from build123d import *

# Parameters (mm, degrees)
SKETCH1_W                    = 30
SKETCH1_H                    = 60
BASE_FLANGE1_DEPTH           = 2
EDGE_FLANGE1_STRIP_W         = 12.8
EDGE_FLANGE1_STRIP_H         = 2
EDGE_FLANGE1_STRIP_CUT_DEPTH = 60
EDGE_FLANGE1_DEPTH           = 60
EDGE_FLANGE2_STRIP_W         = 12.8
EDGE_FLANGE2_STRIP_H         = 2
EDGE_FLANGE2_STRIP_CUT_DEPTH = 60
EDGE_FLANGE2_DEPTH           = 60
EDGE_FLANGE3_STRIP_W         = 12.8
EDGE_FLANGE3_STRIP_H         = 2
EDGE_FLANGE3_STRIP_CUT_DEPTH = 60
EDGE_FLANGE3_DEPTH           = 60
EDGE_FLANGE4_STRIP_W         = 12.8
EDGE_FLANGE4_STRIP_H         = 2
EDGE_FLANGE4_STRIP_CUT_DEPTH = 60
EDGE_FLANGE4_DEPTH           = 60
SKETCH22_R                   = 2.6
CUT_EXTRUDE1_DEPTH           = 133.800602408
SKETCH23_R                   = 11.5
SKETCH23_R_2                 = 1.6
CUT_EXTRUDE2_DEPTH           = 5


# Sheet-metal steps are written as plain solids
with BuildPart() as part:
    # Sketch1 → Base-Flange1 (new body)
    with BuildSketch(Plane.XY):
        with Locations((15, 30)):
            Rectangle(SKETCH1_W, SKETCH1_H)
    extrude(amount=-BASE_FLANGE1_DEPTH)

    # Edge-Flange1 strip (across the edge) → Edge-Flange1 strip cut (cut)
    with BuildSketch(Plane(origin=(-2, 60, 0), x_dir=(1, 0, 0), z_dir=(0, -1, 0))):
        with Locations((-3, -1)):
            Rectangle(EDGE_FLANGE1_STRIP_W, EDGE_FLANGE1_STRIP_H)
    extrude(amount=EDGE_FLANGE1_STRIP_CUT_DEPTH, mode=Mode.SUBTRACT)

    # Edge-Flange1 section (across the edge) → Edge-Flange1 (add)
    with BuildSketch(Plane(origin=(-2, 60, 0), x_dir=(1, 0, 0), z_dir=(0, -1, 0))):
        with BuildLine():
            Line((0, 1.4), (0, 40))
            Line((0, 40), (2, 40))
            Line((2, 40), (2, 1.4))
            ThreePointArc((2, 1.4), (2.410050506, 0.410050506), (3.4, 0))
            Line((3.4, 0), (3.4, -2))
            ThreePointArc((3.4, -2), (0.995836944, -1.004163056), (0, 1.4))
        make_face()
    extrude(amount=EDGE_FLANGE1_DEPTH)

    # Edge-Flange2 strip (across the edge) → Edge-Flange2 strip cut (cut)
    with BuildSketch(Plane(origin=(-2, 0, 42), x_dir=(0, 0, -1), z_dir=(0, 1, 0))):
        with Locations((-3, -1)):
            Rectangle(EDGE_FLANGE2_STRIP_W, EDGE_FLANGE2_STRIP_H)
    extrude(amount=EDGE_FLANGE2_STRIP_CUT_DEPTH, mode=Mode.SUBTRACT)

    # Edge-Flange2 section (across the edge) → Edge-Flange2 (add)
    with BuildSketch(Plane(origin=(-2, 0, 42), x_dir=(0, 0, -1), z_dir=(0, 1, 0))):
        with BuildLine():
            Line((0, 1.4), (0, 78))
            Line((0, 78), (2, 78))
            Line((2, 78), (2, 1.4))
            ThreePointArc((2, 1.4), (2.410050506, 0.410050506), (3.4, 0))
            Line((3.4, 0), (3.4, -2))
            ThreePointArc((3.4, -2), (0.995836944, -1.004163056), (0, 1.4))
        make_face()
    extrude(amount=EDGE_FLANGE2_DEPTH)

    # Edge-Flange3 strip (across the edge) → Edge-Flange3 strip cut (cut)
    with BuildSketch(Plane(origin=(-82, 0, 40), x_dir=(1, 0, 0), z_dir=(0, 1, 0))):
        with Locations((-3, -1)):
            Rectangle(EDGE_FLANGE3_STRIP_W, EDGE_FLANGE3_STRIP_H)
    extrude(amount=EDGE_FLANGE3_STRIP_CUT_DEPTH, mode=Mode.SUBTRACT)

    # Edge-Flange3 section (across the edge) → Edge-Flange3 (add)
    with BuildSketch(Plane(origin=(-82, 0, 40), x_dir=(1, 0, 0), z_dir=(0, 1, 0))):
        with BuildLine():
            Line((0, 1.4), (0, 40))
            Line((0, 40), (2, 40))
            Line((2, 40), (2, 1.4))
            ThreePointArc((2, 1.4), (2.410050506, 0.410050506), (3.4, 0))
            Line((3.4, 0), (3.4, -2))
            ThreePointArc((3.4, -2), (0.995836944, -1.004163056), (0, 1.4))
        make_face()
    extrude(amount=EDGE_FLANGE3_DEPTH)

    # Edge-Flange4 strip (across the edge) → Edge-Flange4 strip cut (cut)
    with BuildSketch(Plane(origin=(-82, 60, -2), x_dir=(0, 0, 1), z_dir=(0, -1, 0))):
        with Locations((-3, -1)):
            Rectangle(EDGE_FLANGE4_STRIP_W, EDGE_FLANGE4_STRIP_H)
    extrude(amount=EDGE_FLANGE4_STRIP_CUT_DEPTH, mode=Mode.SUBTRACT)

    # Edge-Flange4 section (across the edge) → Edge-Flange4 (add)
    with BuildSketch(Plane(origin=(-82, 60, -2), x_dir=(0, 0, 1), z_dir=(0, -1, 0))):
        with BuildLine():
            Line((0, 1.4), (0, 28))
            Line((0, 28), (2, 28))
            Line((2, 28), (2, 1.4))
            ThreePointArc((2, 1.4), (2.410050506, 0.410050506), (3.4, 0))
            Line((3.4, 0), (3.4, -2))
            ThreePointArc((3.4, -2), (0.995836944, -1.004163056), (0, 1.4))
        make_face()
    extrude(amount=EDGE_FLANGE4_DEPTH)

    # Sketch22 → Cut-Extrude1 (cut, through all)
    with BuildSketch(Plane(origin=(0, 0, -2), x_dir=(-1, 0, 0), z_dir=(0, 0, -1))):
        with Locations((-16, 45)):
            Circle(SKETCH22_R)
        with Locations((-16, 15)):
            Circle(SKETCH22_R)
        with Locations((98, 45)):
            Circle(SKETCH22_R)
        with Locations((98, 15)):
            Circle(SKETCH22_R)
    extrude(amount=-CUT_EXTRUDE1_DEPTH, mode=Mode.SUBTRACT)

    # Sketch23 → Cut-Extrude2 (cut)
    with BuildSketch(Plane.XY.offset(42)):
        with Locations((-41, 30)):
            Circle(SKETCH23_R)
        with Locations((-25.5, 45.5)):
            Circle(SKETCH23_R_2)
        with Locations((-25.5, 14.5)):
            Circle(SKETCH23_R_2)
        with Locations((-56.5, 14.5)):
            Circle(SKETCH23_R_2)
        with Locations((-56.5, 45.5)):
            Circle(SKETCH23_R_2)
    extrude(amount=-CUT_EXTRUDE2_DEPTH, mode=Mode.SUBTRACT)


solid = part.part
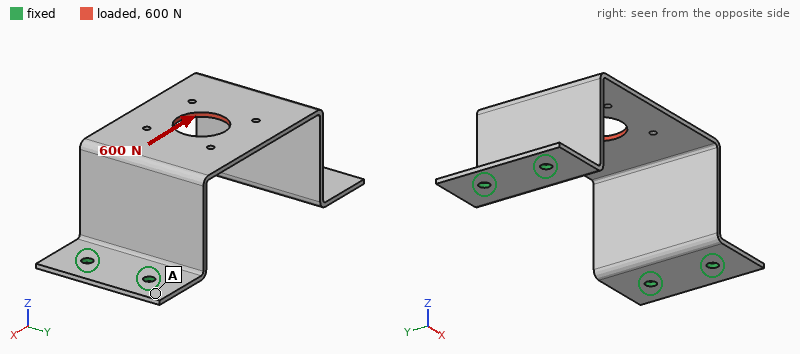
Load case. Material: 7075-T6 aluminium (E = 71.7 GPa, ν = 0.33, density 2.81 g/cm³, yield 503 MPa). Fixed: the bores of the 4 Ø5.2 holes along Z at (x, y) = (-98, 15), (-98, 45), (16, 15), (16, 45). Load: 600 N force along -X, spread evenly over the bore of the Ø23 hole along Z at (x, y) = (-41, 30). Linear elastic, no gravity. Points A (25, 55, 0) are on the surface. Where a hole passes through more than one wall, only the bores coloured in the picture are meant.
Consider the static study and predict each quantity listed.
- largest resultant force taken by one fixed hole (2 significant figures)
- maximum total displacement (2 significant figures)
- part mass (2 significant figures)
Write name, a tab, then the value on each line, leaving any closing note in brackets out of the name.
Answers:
largest resultant force taken by one fixed hole	170 N
maximum total displacement	1.6 mm
part mass	71 g
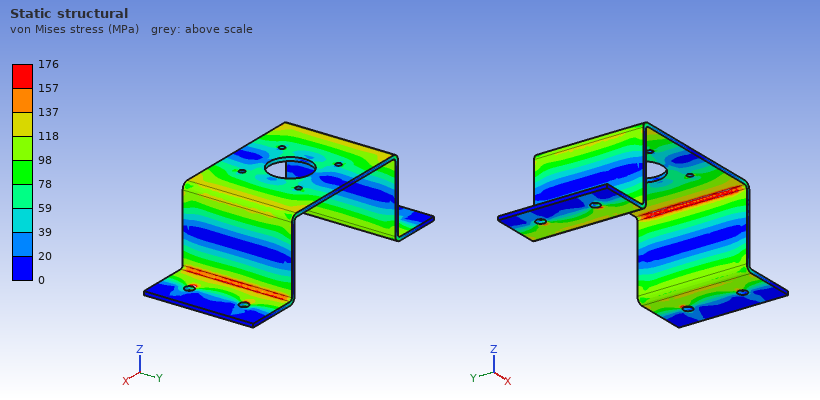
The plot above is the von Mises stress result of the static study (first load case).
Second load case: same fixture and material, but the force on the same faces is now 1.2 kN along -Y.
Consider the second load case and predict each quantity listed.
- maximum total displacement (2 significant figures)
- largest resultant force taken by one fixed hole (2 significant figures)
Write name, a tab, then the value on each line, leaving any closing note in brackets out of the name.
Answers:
maximum total displacement	1.1 mm
largest resultant force taken by one fixed hole	850 N
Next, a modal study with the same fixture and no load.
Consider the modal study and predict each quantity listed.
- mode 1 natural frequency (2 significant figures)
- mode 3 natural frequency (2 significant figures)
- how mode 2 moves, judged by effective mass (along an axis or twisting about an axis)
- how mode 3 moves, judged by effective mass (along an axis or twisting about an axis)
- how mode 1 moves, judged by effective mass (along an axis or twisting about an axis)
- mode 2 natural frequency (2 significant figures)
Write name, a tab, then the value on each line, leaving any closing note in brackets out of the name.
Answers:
mode 1 natural frequency	530 Hz
mode 3 natural frequency	1000 Hz
how mode 2 moves, judged by effective mass	along Y
how mode 3 moves, judged by effective mass	twisting about Z
how mode 1 moves, judged by effective mass	along X
mode 2 natural frequency	890 Hz
